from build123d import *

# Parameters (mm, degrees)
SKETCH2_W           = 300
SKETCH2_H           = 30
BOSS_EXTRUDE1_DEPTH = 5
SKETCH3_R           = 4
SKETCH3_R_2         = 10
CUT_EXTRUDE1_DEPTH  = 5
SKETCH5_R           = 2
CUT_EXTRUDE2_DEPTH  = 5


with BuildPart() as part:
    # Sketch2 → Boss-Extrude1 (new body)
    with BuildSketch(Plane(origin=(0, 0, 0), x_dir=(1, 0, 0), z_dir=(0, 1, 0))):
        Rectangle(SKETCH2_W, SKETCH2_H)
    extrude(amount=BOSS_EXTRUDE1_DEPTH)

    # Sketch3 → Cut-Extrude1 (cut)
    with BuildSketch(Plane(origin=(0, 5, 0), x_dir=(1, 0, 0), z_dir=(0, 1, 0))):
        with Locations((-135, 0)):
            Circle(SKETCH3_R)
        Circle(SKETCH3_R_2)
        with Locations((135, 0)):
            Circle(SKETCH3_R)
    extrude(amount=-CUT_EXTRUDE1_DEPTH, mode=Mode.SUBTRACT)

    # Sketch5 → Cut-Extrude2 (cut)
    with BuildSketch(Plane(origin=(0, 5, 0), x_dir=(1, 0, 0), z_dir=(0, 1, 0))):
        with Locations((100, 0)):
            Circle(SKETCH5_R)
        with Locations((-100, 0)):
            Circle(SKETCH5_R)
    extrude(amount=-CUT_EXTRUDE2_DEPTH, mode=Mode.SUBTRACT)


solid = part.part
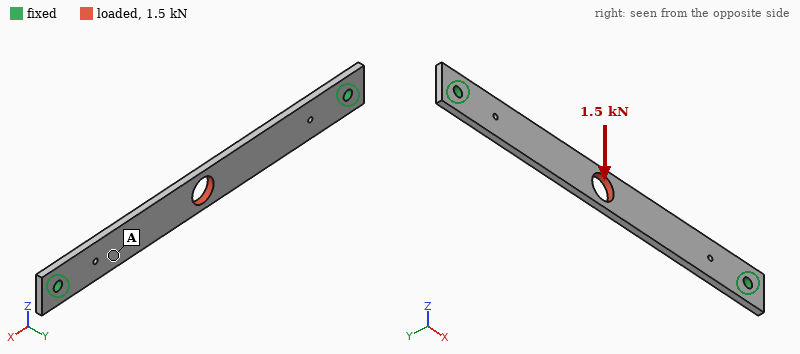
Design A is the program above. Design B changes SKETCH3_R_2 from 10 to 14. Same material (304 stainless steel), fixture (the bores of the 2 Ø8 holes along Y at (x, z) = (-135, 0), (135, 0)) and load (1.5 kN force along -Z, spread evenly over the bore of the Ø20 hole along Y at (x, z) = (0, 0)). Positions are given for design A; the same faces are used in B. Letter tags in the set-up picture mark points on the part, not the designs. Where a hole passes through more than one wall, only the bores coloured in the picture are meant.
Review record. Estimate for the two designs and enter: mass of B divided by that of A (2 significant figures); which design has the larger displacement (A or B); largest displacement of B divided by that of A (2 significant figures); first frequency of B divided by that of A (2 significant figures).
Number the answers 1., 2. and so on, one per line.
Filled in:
1. 0.96
2. B
3. 1.3
4. 0.93
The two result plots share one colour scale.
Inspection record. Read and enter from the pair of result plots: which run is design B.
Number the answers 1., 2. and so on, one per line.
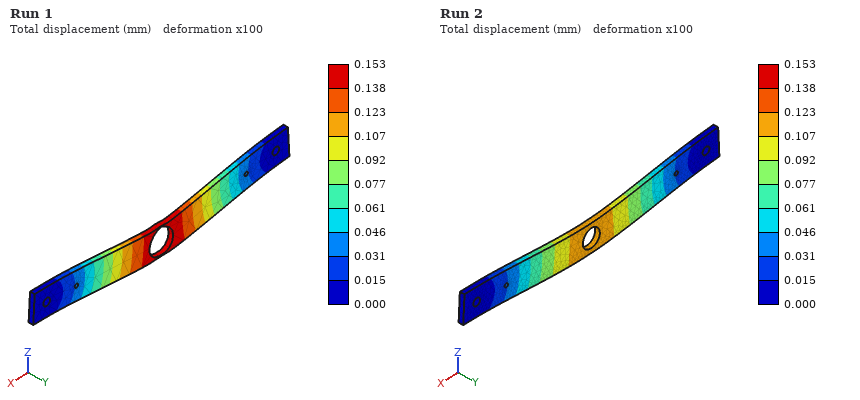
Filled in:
1. Run 1
